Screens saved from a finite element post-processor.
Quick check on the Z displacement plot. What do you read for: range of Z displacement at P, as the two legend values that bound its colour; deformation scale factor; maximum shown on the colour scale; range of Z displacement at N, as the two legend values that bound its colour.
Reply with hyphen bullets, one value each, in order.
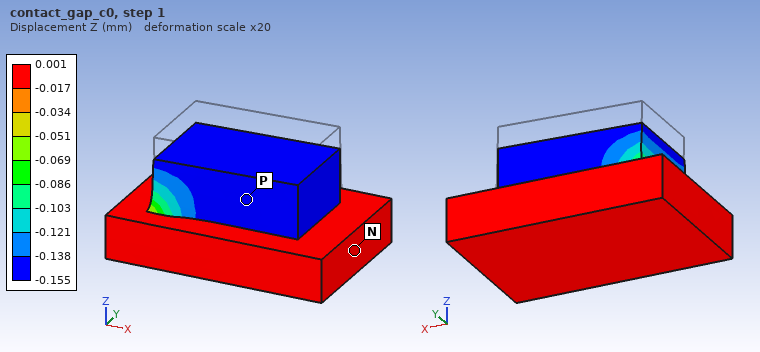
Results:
- -0.155 to -0.138 mm
- 20
- 0.001 mm
- -0.017 to 0.001 mm
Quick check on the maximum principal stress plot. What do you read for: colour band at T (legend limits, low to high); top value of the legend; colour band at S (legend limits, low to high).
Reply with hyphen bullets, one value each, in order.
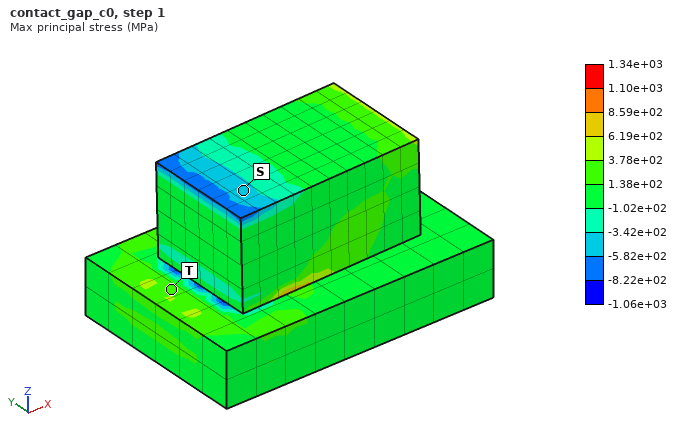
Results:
- 1.38e+02 to 3.78e+02 MPa
- 1.34e+03 MPa
- -5.82e+02 to -3.42e+02 MPa
